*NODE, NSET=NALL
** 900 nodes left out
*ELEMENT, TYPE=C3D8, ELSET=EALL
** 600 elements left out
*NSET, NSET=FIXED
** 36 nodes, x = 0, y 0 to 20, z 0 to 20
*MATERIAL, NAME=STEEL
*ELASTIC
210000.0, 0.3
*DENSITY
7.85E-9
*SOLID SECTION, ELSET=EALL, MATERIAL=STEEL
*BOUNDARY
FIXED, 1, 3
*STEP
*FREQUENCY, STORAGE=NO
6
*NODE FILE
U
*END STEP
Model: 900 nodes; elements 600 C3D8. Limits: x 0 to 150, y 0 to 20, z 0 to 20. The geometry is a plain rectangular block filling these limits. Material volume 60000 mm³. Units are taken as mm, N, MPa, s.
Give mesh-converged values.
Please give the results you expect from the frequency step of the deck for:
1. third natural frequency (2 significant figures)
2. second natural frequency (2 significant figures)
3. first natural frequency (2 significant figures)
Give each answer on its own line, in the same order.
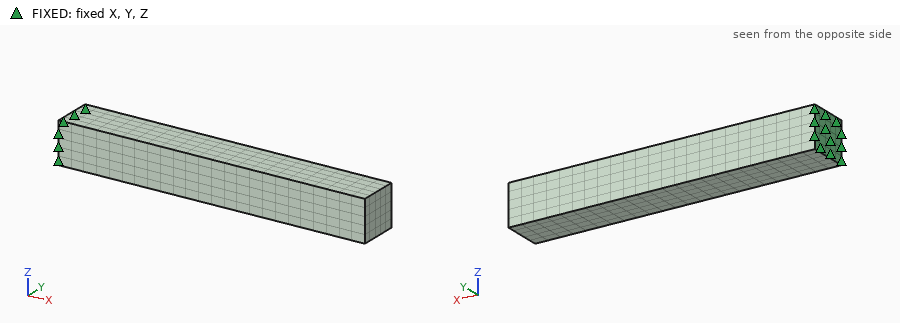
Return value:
4300 Hz
740 Hz
740 Hz
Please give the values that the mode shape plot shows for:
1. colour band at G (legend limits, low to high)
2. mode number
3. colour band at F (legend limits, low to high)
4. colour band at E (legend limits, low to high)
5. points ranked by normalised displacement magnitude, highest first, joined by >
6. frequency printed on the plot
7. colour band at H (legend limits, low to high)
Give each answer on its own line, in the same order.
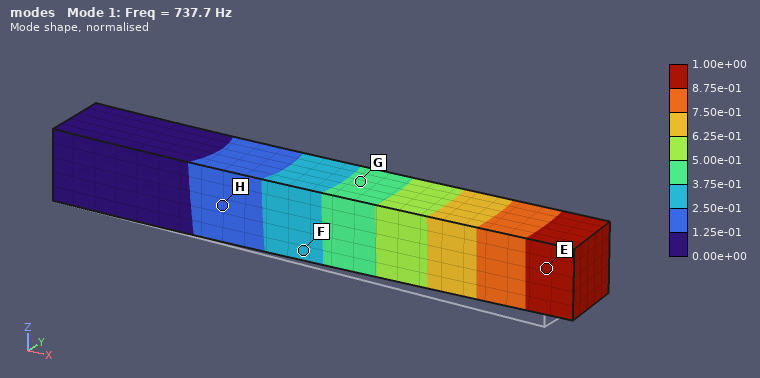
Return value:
3.75e-01 to 5.00e-01
1
2.50e-01 to 3.75e-01
8.75e-01 to 1.00e+00
E > G > F > H
737.7 Hz
1.25e-01 to 2.50e-01
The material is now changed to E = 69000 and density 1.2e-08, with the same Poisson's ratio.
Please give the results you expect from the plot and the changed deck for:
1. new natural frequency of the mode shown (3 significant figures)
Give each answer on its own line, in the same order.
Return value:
342 Hz
